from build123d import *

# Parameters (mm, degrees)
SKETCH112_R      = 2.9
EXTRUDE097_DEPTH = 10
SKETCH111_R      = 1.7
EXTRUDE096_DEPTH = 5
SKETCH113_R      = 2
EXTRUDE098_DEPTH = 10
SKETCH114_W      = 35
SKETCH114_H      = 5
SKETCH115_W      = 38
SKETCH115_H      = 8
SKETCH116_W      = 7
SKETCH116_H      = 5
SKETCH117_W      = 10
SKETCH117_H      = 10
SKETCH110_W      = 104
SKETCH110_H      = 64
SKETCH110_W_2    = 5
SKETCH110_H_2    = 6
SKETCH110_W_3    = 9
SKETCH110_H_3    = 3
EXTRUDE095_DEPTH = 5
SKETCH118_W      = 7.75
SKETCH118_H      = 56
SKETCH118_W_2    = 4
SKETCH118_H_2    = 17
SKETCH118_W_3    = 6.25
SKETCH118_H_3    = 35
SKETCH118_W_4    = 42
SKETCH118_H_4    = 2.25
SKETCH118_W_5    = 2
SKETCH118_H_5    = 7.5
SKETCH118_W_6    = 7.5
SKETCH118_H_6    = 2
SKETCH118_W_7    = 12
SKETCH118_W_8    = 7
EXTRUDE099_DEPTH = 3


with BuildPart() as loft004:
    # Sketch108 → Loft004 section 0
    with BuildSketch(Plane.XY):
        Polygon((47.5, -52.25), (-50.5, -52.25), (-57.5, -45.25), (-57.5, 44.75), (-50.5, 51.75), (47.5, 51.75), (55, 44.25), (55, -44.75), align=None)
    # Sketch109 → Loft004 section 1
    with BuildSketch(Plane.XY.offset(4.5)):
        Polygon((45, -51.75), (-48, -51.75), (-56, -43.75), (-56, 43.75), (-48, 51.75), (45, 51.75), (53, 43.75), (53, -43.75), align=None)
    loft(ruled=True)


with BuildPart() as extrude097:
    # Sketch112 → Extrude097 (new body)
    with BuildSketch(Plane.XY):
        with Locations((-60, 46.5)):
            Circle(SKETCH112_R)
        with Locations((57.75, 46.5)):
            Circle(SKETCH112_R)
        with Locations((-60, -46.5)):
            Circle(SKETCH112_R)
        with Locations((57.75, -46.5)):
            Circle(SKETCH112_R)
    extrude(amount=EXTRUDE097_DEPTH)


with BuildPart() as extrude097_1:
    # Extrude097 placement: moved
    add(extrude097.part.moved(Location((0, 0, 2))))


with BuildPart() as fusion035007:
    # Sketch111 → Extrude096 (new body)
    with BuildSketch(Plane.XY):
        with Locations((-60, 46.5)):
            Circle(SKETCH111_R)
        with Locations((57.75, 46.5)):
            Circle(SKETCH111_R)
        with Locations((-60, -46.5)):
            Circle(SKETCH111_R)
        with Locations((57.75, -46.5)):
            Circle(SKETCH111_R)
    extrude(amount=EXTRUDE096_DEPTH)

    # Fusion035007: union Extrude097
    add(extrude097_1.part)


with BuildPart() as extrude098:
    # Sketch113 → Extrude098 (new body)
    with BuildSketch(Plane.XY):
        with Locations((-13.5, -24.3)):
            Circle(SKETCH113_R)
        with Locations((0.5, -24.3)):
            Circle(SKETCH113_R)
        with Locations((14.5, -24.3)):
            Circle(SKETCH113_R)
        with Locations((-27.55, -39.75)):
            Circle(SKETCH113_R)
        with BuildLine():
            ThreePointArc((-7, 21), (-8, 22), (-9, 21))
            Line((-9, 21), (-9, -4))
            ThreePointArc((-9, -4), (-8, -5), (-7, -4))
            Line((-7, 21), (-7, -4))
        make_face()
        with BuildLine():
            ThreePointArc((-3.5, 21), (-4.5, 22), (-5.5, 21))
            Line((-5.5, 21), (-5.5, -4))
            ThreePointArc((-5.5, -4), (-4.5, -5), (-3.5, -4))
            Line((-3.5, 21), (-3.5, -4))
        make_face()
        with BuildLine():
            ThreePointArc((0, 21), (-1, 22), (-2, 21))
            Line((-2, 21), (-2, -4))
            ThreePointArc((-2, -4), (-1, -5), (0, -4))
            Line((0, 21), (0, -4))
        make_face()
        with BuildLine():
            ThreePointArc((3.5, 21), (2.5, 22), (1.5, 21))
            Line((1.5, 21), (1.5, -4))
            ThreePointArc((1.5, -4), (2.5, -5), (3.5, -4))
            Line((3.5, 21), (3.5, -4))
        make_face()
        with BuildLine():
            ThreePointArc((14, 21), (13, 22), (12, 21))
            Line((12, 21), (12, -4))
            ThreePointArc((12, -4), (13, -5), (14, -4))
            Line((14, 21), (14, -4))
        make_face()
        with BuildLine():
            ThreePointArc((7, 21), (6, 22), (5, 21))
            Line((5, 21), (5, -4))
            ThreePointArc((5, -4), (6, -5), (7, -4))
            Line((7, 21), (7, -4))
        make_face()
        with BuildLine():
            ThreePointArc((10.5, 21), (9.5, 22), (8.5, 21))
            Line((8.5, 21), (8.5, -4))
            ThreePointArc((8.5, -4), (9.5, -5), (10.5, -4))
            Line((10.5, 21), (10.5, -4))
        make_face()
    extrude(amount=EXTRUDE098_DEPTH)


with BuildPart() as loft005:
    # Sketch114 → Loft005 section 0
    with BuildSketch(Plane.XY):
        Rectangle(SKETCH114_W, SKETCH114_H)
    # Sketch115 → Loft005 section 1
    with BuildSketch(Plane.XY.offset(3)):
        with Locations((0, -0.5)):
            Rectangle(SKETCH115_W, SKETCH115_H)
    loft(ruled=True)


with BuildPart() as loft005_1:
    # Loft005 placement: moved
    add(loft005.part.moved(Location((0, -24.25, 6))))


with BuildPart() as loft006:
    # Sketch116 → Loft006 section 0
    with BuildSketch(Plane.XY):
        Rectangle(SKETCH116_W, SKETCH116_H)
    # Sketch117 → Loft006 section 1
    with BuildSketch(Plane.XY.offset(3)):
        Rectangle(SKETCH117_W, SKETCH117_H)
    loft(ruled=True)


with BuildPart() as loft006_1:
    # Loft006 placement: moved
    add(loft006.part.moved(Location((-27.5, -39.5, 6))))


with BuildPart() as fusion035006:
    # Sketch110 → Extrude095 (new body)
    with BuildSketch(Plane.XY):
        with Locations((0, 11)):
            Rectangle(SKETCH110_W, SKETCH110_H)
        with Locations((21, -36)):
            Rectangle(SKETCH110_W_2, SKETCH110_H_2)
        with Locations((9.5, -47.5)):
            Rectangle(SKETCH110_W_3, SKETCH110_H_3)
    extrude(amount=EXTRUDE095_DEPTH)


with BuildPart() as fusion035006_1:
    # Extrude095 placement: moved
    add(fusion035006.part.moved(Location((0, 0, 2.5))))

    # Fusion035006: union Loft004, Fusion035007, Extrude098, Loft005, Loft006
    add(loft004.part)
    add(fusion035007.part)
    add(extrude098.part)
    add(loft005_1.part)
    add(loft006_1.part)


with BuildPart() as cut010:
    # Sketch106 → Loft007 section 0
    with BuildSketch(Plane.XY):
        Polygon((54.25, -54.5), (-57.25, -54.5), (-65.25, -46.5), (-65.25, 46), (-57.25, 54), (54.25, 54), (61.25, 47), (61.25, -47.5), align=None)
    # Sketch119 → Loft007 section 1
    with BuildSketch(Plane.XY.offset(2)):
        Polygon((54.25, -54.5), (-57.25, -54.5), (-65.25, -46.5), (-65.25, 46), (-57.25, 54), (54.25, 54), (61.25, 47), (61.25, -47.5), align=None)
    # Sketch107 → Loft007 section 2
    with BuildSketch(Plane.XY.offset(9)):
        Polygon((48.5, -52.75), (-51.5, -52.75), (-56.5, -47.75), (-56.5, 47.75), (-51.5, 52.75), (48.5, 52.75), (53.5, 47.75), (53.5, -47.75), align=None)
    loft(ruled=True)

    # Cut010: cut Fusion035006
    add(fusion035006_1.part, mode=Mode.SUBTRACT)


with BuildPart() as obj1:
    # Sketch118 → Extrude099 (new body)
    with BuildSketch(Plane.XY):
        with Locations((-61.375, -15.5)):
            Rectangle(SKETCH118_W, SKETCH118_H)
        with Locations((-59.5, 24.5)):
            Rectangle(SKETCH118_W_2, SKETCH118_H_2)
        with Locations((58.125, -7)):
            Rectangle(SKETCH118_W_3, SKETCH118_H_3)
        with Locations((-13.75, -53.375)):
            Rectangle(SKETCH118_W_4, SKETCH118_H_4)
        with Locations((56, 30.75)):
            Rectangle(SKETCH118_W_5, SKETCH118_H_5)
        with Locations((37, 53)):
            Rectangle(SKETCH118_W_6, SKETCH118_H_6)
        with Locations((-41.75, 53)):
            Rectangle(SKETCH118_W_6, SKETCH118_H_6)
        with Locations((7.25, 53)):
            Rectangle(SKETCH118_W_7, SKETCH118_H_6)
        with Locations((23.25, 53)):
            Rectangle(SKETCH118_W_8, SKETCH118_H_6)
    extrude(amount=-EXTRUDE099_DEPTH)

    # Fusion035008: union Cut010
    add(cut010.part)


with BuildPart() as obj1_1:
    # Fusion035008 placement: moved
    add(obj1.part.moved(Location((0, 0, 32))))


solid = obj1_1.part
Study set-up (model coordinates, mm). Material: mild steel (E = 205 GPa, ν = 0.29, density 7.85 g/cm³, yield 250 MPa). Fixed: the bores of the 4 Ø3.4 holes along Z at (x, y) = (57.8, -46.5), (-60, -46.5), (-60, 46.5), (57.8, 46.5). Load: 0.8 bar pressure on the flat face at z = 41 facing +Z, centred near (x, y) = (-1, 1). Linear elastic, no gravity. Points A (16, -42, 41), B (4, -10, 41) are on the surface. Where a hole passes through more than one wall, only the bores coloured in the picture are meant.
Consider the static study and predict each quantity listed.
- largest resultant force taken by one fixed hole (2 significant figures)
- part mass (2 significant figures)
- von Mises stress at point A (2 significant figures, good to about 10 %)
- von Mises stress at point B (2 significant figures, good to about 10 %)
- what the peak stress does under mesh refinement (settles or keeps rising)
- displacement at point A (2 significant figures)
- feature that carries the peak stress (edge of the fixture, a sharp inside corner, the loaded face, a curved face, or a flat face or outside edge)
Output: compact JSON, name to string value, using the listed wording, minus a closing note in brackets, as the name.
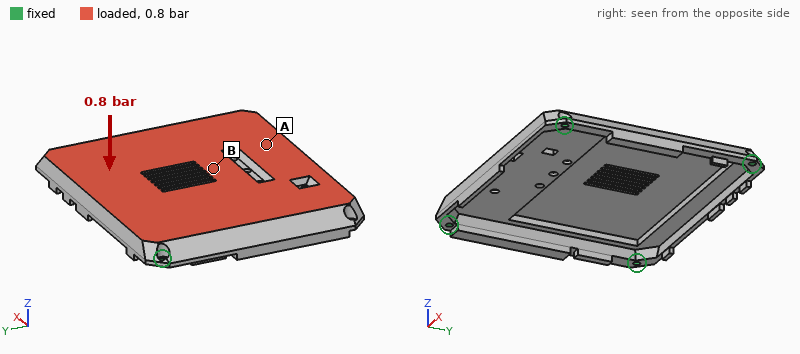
{"largest resultant force taken by one fixed hole": "700 N", "part mass": "350 g", "von Mises stress at point A": "18 MPa", "von Mises stress at point B": "32 MPa", "what the peak stress does under mesh refinement": "keeps rising", "displacement at point A": "0.027 mm", "feature that carries the peak stress": "edge of the fixture"}
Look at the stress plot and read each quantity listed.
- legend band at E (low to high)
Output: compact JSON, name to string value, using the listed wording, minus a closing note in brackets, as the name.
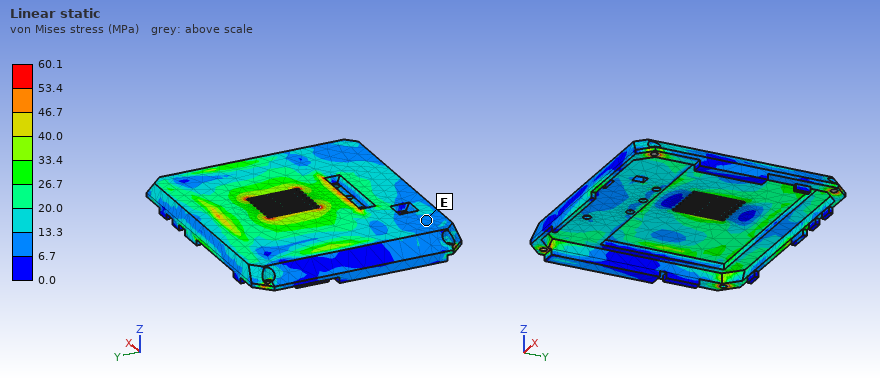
{"legend band at E": "6.7 to 13.3 MPa"}
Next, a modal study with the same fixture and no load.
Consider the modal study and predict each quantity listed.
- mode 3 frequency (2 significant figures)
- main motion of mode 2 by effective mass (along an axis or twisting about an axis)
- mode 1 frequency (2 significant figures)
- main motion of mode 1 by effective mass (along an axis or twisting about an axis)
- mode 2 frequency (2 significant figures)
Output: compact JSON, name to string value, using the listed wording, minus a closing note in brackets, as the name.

{"mode 3 frequency": "2500 Hz", "main motion of mode 2 by effective mass": "twisting about X", "mode 1 frequency": "1400 Hz", "main motion of mode 1 by effective mass": "along Z", "mode 2 frequency": "1900 Hz"}
